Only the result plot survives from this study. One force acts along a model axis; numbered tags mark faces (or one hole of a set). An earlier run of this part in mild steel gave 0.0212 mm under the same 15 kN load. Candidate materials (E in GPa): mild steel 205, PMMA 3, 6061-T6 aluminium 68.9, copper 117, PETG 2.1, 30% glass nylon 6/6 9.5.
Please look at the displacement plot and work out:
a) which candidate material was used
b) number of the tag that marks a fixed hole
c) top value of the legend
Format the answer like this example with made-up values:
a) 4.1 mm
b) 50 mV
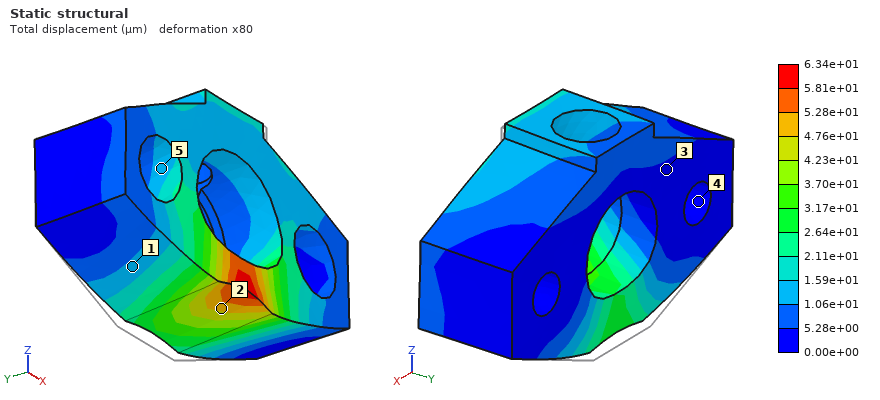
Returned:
a) 6061-T6 aluminium
b) 4
c) 6.34e+01 µm
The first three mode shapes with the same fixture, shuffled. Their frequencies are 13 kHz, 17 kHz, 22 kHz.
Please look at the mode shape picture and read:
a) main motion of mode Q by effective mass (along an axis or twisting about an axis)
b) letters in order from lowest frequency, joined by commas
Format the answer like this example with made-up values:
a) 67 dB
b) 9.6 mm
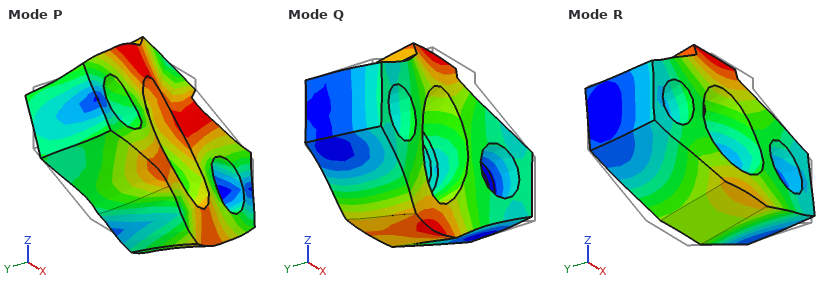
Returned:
a) along Y
b) R, Q, P
